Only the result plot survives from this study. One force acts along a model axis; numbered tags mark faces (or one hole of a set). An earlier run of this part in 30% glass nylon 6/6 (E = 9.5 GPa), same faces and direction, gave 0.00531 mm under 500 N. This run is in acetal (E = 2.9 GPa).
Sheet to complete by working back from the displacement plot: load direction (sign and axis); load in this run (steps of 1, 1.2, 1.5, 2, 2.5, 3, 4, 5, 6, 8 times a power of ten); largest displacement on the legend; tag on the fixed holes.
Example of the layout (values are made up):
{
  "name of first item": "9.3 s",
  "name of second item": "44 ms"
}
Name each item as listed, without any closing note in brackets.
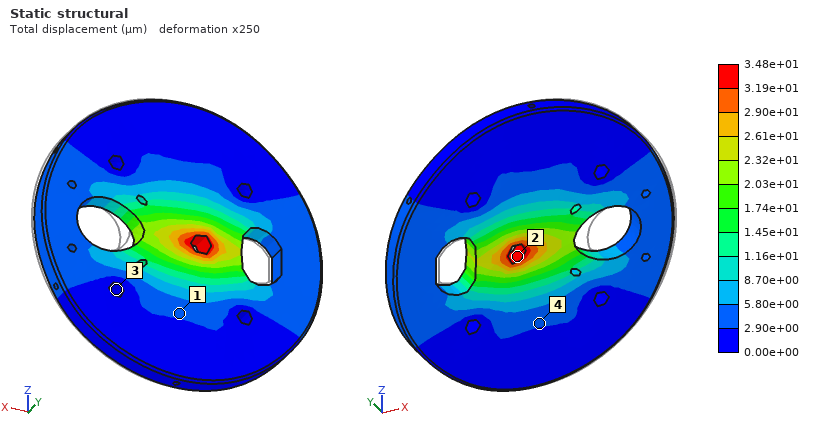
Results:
{
  "load direction": "-X",
  "load in this run": "1 kN",
  "largest displacement on the legend": "3.48e+01 µm",
  "tag on the fixed holes": "3"
}
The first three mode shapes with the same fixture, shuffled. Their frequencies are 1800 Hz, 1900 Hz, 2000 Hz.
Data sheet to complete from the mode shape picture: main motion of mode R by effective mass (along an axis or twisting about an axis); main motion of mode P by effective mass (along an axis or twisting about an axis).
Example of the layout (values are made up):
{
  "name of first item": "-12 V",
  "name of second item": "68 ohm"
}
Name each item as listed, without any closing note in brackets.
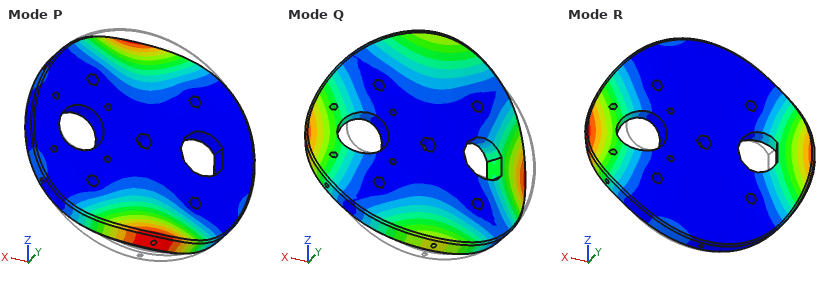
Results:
{
  "main motion of mode R by effective mass": "twisting about Z",
  "main motion of mode P by effective mass": "twisting about X"
}
